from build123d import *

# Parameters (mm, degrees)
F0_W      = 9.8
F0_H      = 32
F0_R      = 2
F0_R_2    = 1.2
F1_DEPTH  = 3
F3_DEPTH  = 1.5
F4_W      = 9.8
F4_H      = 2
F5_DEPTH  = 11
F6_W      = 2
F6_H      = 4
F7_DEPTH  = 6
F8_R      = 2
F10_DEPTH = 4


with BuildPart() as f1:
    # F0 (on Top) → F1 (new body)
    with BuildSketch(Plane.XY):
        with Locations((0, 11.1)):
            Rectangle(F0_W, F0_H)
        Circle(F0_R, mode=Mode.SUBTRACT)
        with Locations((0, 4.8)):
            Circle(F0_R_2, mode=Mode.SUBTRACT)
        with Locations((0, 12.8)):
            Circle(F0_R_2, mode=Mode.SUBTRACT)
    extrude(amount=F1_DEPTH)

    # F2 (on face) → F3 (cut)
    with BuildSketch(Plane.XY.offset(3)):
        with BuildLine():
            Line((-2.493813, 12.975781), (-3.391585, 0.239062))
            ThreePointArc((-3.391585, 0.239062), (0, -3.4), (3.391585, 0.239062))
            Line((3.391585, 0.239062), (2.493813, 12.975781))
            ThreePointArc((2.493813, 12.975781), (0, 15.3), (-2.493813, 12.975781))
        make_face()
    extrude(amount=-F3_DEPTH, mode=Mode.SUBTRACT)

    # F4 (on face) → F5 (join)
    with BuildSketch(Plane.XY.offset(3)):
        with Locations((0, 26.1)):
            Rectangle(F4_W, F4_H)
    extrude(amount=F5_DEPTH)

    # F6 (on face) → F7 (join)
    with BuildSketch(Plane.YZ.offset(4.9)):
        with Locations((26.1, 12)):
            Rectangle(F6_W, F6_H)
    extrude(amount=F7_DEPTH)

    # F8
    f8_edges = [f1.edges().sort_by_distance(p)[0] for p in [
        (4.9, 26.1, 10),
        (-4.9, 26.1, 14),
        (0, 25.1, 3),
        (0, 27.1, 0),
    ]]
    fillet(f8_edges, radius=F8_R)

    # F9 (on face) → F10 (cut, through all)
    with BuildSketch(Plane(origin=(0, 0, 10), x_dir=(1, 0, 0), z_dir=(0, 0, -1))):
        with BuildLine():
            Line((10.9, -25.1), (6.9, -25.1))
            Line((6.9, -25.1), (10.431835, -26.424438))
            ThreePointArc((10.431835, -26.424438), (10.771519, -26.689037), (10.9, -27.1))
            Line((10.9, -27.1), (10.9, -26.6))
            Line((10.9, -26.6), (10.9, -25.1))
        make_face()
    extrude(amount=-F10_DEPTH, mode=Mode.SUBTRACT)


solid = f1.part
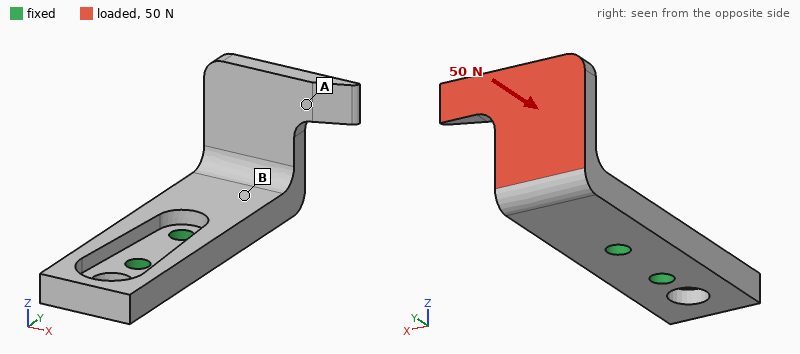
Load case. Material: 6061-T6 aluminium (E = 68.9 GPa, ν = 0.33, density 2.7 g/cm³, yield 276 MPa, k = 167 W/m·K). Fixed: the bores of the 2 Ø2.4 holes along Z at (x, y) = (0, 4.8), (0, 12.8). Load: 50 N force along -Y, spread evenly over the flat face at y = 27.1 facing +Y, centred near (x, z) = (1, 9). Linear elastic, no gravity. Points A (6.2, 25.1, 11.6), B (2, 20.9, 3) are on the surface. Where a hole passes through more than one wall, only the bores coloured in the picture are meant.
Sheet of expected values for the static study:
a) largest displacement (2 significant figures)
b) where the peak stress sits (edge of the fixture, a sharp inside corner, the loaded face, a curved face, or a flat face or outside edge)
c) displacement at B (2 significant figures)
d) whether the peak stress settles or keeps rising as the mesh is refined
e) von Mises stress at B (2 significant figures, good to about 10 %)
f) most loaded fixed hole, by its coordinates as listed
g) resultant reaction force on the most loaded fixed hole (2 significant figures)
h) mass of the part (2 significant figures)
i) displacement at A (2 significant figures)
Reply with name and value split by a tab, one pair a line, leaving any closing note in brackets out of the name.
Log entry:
largest displacement	87 µm
where the peak stress sits	edge of the fixture
displacement at B	15 µm
whether the peak stress settles or keeps rising as the mesh is refined	keeps rising
von Mises stress at B	26 MPa
most loaded fixed hole, by its coordinates as listed	(0, 4.8)
resultant reaction force on the most loaded fixed hole	56 N
mass of the part	2.7 g
displacement at A	63 µm
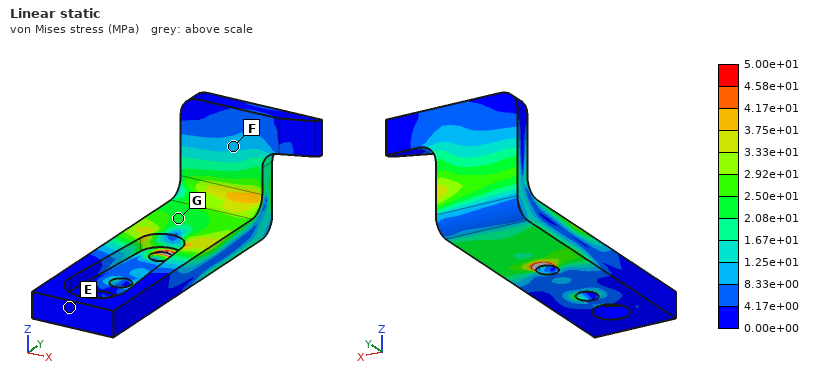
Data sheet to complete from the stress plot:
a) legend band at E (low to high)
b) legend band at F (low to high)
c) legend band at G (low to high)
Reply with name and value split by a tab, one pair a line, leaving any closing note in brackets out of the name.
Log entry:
legend band at E	0.00e+00 to 4.17e+00 MPa
legend band at F	8.33e+00 to 1.25e+01 MPa
legend band at G	2.08e+01 to 2.50e+01 MPa
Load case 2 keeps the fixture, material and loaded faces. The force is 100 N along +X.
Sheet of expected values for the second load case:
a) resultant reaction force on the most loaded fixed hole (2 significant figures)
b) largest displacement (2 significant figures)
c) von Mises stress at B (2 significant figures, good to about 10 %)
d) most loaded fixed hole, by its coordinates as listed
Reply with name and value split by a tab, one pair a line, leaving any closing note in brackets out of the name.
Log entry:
resultant reaction force on the most loaded fixed hole	210 N
largest displacement	0.13 mm
von Mises stress at B	55 MPa
most loaded fixed hole, by its coordinates as listed	(0, 12.8)
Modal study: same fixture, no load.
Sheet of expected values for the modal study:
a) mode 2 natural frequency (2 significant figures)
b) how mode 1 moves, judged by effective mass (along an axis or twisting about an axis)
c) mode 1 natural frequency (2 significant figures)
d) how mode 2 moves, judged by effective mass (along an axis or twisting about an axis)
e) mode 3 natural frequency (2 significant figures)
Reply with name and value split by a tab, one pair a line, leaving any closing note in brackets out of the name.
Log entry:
mode 2 natural frequency	6200 Hz
how mode 1 moves, judged by effective mass	along Z
mode 1 natural frequency	4300 Hz
how mode 2 moves, judged by effective mass	along X
mode 3 natural frequency	11 kHz
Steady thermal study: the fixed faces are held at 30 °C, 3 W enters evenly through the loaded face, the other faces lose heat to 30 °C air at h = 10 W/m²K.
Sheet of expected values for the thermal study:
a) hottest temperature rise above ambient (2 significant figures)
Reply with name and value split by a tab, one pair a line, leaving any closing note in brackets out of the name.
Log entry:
hottest temperature rise above ambient	16 K
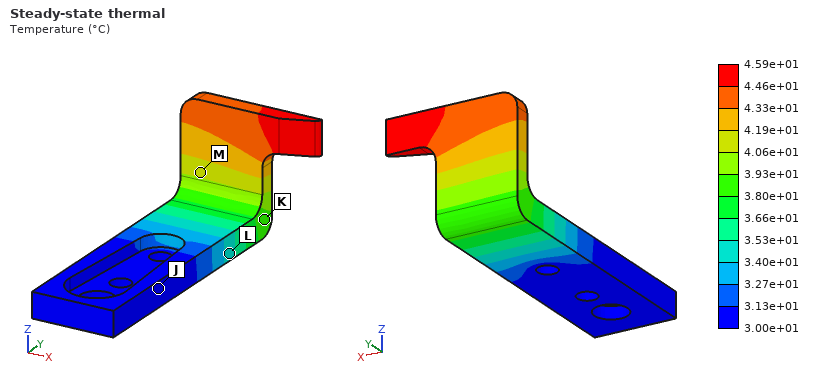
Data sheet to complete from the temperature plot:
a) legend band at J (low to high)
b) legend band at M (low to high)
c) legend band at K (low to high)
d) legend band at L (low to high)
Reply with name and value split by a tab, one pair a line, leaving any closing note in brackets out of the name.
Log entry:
legend band at J	3.00e+01 to 3.13e+01 °C
legend band at M	4.06e+01 to 4.19e+01 °C
legend band at K	3.80e+01 to 3.93e+01 °C
legend band at L	3.40e+01 to 3.53e+01 °C
